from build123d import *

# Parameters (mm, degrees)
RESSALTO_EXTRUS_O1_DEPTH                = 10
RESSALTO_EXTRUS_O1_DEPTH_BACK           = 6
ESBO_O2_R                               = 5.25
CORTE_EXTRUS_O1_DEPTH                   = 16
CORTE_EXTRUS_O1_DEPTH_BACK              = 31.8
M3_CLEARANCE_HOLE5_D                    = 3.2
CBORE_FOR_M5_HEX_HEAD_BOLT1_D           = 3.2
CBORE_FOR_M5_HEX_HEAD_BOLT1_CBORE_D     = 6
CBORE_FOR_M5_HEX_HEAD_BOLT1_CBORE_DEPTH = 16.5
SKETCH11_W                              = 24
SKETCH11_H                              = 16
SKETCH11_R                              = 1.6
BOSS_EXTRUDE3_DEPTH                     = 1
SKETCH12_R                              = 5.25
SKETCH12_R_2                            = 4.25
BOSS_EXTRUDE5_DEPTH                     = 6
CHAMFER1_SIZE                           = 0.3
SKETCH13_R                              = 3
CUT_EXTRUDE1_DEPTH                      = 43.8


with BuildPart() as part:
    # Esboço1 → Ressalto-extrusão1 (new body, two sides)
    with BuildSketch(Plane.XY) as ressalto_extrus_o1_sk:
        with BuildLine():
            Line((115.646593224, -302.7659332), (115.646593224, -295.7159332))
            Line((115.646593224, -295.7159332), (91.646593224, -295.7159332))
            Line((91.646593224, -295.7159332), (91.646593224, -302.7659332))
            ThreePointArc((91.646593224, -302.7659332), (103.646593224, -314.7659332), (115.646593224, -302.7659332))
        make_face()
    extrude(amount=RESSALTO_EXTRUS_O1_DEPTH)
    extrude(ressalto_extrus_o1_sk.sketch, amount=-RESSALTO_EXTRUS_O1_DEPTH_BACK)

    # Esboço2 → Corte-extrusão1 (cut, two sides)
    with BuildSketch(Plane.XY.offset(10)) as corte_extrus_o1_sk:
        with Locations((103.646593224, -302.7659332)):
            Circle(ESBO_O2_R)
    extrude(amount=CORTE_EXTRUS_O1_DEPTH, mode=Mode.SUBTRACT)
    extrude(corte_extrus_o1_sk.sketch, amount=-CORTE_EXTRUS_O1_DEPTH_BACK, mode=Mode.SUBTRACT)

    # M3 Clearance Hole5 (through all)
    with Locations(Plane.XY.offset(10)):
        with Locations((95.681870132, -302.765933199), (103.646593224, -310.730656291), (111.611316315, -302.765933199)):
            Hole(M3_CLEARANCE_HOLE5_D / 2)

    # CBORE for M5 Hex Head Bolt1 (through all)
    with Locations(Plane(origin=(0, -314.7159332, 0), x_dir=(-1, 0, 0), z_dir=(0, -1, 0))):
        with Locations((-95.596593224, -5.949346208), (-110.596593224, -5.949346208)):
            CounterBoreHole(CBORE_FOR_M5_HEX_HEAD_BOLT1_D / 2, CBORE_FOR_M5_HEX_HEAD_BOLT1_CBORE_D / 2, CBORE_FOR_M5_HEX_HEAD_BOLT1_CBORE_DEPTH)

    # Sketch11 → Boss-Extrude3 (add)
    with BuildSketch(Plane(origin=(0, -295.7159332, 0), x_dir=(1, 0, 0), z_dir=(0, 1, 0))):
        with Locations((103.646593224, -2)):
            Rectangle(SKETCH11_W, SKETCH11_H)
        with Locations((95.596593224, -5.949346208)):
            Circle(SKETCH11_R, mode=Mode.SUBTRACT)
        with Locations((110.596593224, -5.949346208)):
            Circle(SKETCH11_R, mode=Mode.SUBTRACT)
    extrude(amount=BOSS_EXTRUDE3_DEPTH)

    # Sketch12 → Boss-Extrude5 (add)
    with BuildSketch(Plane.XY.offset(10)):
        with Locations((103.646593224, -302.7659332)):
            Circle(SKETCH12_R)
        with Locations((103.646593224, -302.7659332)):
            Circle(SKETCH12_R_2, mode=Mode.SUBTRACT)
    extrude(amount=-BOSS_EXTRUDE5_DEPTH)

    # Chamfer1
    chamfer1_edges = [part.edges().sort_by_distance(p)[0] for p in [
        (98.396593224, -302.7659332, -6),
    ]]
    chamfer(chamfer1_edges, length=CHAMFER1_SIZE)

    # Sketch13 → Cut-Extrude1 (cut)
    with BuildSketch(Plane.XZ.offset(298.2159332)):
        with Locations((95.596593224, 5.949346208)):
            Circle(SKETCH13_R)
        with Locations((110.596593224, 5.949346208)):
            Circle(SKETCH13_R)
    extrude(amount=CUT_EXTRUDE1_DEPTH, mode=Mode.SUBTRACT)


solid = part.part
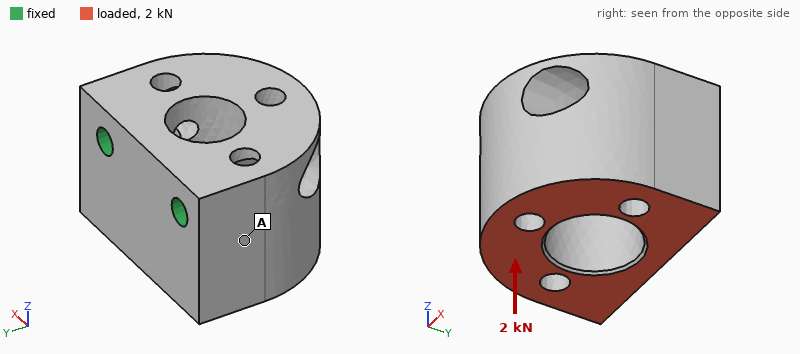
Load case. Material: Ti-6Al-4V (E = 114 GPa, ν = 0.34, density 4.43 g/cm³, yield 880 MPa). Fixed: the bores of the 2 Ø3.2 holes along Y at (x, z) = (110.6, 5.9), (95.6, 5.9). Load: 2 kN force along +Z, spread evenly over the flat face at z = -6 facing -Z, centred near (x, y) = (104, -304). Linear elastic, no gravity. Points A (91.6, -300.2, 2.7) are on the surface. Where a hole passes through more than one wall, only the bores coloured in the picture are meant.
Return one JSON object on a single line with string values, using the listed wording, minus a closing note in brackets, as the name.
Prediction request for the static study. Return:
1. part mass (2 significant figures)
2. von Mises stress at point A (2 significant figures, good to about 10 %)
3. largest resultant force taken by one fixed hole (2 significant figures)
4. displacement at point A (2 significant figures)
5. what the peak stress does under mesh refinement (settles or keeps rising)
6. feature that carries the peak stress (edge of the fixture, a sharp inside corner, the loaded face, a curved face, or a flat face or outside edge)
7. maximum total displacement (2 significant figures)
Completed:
{"part mass": "19 g", "von Mises stress at point A": "34 MPa", "largest resultant force taken by one fixed hole": "1.0 kN", "displacement at point A": "11 µm", "what the peak stress does under mesh refinement": "keeps rising", "feature that carries the peak stress": "edge of the fixture", "maximum total displacement": "55 µm"}
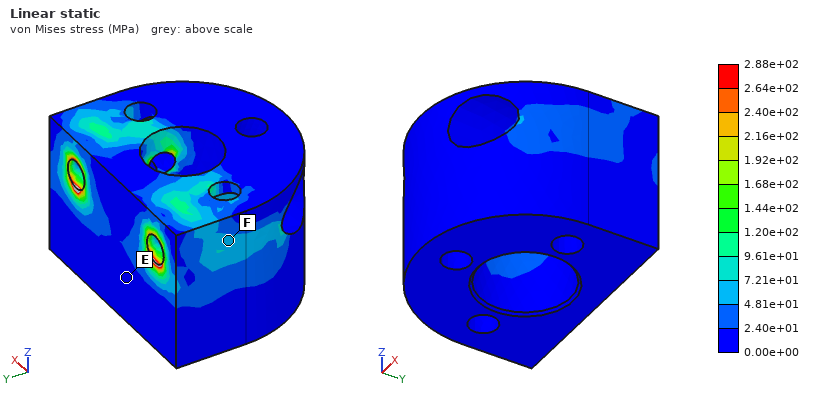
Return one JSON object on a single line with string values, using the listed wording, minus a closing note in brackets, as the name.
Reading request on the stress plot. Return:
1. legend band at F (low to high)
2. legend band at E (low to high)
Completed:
{"legend band at F": "4.81e+01 to 7.21e+01 MPa", "legend band at E": "0.00e+00 to 2.40e+01 MPa"}
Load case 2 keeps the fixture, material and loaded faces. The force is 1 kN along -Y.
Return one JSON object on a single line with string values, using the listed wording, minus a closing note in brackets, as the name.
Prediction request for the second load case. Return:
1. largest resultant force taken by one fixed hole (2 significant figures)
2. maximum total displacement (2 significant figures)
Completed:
{"largest resultant force taken by one fixed hole": "520 N", "maximum total displacement": "43 µm"}
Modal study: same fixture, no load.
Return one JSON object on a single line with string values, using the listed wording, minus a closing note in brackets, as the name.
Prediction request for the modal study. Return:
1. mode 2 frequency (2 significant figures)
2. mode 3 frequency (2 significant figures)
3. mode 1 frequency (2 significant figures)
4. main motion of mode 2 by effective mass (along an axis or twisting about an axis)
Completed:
{"mode 2 frequency": "15 kHz", "mode 3 frequency": "24 kHz", "mode 1 frequency": "7900 Hz", "main motion of mode 2 by effective mass": "along X"}
